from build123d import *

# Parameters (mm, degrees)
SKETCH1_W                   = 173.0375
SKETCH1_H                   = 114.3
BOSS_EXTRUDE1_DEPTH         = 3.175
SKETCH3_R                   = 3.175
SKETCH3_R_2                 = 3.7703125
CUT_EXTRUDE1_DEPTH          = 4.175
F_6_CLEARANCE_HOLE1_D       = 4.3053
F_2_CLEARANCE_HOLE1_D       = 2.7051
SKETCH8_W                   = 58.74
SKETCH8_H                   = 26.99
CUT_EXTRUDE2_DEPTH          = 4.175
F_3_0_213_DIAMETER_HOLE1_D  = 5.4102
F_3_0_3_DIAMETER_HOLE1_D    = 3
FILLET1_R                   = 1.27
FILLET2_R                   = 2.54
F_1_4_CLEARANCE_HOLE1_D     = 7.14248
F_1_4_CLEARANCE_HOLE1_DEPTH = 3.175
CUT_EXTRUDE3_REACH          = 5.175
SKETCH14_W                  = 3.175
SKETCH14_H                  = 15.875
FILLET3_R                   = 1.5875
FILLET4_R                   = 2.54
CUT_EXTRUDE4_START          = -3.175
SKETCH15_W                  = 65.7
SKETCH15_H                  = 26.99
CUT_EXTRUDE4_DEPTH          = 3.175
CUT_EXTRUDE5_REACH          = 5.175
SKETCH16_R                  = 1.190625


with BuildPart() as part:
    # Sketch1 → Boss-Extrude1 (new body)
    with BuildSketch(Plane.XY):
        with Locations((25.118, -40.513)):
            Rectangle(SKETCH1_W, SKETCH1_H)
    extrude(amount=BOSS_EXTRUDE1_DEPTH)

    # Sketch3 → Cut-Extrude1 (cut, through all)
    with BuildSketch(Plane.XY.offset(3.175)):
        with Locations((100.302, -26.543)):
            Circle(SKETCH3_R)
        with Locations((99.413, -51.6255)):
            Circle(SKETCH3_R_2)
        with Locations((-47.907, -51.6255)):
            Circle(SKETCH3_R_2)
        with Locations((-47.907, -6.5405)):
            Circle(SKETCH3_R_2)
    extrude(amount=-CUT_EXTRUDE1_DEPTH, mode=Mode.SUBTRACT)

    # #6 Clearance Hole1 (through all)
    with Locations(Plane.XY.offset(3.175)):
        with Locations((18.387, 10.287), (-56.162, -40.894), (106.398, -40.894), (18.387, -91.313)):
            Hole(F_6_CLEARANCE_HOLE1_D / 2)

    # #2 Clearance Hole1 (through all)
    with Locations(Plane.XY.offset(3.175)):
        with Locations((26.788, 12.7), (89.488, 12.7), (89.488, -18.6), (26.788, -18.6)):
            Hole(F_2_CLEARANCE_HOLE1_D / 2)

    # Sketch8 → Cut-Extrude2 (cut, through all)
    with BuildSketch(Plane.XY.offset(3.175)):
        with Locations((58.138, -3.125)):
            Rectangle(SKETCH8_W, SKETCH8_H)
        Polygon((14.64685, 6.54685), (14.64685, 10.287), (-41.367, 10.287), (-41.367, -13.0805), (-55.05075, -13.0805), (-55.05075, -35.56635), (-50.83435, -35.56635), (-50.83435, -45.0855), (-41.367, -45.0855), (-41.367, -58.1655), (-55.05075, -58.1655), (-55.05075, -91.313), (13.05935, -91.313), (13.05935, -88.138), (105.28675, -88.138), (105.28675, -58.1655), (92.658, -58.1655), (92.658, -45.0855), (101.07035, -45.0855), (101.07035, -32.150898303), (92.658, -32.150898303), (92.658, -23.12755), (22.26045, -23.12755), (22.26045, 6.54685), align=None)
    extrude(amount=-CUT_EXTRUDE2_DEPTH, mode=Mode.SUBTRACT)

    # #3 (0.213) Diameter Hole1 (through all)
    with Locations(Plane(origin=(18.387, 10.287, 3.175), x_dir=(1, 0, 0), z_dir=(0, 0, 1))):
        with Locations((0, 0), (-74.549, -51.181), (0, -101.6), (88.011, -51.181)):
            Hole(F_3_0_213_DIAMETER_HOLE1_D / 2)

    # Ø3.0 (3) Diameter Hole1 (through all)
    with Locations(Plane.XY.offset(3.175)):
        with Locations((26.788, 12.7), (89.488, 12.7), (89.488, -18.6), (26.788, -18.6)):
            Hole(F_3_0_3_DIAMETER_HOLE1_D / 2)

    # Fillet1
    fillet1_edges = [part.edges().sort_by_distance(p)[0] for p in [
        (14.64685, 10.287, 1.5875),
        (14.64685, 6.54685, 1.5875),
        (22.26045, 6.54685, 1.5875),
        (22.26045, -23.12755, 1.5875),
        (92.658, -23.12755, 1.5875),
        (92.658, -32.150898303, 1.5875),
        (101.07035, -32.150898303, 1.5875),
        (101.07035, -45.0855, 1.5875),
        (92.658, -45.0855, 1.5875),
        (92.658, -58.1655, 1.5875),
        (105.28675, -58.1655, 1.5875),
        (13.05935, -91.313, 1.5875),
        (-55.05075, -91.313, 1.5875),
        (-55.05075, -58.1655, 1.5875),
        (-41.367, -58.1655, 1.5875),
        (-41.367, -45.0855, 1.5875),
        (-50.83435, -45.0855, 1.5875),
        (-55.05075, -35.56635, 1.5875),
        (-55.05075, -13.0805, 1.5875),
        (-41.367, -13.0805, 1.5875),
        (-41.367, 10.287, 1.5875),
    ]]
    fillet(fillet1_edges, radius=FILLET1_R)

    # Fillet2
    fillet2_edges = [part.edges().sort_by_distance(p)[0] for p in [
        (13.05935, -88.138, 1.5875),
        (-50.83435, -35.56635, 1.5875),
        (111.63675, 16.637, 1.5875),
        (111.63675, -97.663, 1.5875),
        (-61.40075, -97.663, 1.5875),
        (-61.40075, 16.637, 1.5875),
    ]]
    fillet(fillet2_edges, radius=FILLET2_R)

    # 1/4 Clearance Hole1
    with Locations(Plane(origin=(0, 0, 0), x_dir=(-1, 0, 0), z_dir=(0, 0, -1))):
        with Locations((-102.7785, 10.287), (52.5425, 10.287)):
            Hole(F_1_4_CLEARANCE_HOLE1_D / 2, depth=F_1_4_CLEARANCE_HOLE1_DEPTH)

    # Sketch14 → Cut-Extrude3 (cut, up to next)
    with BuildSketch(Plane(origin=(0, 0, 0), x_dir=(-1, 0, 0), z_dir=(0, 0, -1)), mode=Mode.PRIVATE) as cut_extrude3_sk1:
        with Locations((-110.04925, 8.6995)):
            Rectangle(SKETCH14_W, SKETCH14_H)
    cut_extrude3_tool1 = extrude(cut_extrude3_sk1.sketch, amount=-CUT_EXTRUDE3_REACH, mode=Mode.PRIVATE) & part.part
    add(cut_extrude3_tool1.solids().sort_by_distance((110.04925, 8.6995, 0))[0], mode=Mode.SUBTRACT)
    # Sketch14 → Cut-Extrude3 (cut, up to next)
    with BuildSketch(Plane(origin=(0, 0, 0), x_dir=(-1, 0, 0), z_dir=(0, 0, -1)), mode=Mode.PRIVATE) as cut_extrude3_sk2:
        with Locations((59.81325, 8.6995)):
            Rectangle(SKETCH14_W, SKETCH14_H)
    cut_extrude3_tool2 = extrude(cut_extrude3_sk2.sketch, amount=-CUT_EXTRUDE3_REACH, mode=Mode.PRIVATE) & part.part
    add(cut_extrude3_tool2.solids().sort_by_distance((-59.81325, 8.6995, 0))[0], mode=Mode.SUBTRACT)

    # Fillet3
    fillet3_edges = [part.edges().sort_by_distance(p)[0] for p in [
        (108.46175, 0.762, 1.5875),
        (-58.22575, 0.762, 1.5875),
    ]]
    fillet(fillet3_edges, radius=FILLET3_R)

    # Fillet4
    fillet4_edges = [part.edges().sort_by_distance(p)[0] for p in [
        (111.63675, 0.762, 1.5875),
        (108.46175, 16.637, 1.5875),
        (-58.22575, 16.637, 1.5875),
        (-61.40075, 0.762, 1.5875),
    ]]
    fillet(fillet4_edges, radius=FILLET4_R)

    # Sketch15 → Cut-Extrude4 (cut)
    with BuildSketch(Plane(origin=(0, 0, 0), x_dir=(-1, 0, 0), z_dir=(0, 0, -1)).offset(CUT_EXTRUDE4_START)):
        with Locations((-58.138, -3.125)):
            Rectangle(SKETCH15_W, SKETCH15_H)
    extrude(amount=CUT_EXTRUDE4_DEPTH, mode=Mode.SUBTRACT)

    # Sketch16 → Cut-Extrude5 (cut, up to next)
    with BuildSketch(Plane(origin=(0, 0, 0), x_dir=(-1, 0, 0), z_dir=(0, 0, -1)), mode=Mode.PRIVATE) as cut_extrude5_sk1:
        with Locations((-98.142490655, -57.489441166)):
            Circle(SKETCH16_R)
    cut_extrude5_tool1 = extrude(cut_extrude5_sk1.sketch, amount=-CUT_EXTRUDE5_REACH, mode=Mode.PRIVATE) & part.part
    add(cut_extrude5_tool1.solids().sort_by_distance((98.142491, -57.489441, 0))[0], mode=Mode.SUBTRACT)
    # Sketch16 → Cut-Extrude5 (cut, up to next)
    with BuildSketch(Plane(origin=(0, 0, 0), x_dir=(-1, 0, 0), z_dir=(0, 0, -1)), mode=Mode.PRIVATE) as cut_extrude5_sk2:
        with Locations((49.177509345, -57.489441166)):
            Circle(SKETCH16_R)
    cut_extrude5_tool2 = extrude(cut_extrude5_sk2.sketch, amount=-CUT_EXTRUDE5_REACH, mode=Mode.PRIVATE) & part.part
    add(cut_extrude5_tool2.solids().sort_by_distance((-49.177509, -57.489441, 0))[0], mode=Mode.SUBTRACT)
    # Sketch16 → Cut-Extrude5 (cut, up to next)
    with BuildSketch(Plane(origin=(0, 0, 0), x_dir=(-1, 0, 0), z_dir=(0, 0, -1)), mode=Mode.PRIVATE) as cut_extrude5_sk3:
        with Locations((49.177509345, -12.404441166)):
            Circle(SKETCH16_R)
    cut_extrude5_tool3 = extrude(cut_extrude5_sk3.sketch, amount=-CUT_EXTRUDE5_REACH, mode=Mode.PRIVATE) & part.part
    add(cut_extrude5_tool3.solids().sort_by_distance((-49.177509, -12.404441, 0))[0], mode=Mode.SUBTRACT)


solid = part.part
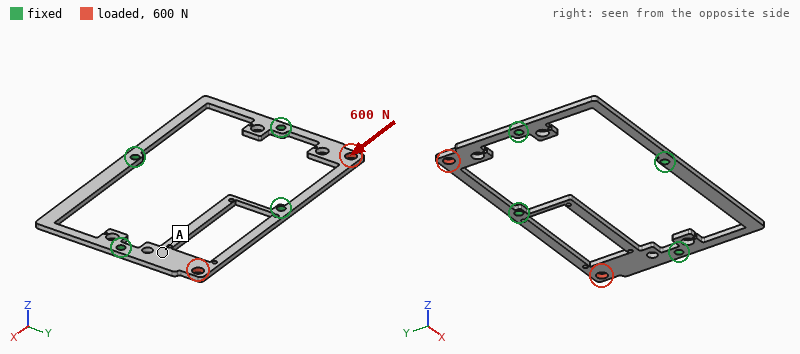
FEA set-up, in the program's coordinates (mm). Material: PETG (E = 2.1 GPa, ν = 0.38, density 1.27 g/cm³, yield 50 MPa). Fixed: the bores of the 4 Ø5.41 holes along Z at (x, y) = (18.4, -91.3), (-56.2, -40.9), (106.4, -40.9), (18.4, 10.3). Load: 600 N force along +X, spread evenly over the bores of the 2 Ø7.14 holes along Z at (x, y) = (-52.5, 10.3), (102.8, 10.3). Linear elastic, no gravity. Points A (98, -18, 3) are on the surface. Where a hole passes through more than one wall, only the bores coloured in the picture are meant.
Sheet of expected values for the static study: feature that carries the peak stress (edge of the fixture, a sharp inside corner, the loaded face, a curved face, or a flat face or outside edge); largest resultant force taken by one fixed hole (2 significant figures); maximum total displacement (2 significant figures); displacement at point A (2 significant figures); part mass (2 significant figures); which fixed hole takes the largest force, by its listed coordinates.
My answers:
a curved face
540 N
0.63 mm
0.26 mm
21 g
(18.4, 10.3)
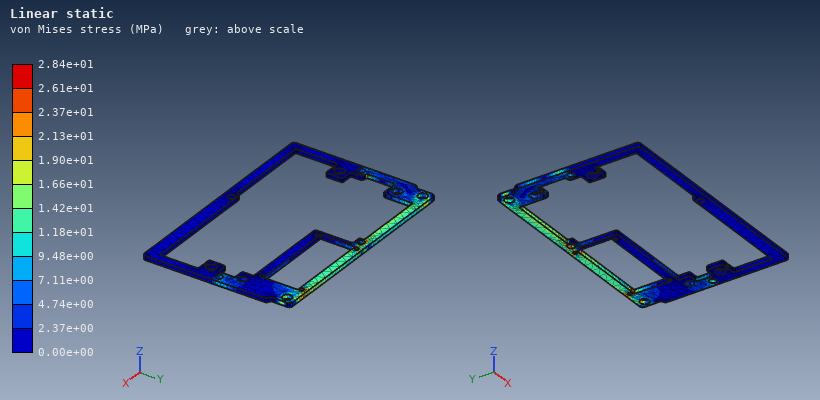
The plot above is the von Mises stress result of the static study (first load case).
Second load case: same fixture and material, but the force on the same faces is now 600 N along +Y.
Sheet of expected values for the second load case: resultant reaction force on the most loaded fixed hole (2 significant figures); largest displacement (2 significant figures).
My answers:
300 N
0.65 mm
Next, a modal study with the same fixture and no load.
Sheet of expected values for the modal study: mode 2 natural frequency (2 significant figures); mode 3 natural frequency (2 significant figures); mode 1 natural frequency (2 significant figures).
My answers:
200 Hz
210 Hz
200 Hz
